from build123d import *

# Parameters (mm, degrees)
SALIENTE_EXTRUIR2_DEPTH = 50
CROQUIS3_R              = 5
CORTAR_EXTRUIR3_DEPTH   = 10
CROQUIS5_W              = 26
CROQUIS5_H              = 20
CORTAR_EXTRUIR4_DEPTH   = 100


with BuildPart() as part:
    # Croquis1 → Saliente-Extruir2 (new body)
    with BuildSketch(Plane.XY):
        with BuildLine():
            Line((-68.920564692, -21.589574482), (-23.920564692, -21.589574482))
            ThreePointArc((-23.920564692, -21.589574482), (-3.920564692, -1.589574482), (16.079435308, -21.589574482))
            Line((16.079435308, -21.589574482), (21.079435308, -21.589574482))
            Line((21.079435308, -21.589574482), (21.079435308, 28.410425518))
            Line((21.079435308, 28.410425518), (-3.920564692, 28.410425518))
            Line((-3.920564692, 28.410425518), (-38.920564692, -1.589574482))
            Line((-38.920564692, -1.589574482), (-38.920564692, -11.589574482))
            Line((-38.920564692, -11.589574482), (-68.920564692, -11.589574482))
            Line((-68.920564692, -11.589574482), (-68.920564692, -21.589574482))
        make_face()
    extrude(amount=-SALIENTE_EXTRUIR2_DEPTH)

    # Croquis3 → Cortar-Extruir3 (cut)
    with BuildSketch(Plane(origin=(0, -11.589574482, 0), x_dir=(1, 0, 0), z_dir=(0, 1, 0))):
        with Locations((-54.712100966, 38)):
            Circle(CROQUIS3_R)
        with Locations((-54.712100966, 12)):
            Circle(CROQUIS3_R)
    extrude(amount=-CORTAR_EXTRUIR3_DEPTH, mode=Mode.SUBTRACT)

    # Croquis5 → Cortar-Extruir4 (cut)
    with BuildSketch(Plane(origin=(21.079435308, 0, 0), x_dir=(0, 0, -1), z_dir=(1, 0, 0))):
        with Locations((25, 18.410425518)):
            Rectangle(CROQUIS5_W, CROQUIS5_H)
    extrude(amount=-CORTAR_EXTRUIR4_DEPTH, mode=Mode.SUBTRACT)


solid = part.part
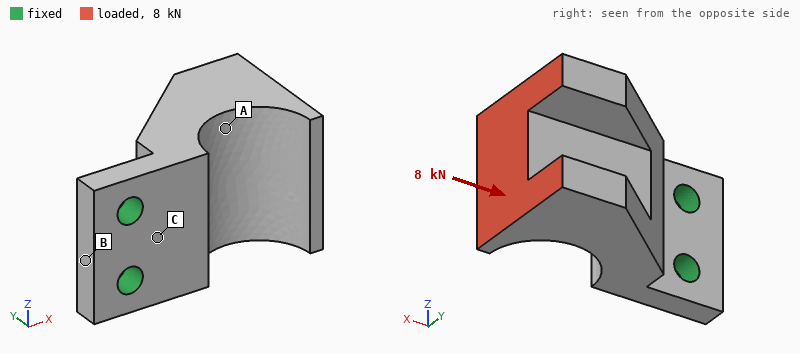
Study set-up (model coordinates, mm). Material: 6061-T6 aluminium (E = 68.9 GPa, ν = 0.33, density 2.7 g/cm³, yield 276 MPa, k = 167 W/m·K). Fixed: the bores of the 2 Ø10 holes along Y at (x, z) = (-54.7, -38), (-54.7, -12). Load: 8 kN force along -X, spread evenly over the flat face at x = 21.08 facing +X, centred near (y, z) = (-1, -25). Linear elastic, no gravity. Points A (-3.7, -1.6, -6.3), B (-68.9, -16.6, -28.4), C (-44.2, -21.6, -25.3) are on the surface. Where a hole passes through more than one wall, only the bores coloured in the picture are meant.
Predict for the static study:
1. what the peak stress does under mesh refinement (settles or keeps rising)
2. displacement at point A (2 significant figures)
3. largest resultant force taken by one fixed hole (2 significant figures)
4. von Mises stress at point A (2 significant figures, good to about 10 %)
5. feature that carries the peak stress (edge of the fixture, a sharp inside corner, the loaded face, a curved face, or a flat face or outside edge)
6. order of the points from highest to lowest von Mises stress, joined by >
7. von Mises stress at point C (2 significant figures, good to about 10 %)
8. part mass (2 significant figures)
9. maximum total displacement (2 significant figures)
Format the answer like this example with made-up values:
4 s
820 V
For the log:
keeps rising
0.33 mm
4.1 kN
37 MPa
edge of the fixture
C > A > B
110 MPa
230 g
0.60 mm
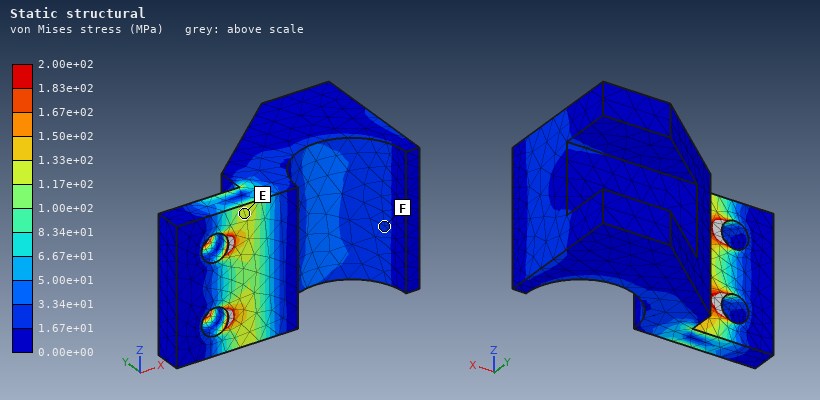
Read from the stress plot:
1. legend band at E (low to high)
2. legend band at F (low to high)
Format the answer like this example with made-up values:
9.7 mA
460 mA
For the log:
1.17e+02 to 1.33e+02 MPa
1.67e+01 to 3.34e+01 MPa
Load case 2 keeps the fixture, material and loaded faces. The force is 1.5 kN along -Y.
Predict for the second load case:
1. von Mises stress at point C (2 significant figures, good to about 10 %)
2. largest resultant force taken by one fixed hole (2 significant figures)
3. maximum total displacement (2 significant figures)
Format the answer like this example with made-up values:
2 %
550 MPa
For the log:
93 MPa
760 N
0.54 mm
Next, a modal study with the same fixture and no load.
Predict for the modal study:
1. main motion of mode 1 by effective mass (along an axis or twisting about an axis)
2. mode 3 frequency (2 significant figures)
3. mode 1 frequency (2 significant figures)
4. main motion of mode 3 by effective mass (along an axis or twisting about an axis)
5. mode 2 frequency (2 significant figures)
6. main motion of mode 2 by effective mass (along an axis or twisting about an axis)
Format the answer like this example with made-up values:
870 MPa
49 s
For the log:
along Y
3200 Hz
950 Hz
twisting about X
2800 Hz
along Z
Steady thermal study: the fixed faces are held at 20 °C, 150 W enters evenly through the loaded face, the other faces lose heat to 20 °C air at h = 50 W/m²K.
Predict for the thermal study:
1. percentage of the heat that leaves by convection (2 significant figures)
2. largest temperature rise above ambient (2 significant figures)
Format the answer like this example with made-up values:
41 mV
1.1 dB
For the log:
24 %
84 K
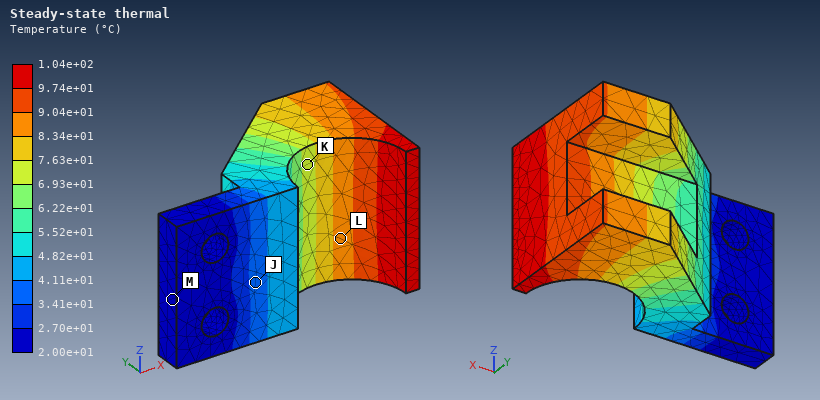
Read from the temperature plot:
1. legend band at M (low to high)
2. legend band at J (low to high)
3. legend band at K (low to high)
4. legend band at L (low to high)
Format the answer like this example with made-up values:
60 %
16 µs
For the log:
2.00e+01 to 2.70e+01 °C
3.41e+01 to 4.11e+01 °C
6.93e+01 to 7.63e+01 °C
8.34e+01 to 9.04e+01 °C
